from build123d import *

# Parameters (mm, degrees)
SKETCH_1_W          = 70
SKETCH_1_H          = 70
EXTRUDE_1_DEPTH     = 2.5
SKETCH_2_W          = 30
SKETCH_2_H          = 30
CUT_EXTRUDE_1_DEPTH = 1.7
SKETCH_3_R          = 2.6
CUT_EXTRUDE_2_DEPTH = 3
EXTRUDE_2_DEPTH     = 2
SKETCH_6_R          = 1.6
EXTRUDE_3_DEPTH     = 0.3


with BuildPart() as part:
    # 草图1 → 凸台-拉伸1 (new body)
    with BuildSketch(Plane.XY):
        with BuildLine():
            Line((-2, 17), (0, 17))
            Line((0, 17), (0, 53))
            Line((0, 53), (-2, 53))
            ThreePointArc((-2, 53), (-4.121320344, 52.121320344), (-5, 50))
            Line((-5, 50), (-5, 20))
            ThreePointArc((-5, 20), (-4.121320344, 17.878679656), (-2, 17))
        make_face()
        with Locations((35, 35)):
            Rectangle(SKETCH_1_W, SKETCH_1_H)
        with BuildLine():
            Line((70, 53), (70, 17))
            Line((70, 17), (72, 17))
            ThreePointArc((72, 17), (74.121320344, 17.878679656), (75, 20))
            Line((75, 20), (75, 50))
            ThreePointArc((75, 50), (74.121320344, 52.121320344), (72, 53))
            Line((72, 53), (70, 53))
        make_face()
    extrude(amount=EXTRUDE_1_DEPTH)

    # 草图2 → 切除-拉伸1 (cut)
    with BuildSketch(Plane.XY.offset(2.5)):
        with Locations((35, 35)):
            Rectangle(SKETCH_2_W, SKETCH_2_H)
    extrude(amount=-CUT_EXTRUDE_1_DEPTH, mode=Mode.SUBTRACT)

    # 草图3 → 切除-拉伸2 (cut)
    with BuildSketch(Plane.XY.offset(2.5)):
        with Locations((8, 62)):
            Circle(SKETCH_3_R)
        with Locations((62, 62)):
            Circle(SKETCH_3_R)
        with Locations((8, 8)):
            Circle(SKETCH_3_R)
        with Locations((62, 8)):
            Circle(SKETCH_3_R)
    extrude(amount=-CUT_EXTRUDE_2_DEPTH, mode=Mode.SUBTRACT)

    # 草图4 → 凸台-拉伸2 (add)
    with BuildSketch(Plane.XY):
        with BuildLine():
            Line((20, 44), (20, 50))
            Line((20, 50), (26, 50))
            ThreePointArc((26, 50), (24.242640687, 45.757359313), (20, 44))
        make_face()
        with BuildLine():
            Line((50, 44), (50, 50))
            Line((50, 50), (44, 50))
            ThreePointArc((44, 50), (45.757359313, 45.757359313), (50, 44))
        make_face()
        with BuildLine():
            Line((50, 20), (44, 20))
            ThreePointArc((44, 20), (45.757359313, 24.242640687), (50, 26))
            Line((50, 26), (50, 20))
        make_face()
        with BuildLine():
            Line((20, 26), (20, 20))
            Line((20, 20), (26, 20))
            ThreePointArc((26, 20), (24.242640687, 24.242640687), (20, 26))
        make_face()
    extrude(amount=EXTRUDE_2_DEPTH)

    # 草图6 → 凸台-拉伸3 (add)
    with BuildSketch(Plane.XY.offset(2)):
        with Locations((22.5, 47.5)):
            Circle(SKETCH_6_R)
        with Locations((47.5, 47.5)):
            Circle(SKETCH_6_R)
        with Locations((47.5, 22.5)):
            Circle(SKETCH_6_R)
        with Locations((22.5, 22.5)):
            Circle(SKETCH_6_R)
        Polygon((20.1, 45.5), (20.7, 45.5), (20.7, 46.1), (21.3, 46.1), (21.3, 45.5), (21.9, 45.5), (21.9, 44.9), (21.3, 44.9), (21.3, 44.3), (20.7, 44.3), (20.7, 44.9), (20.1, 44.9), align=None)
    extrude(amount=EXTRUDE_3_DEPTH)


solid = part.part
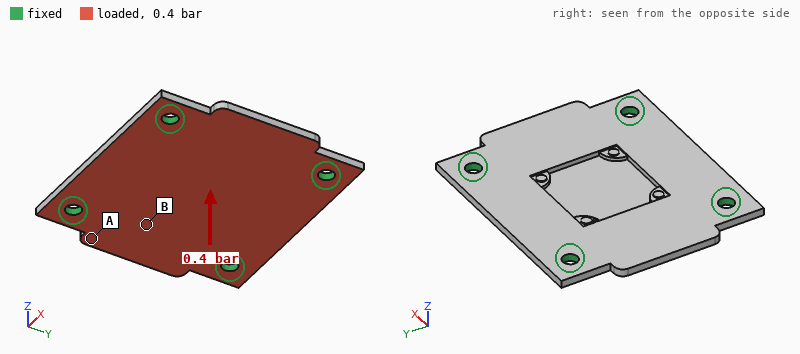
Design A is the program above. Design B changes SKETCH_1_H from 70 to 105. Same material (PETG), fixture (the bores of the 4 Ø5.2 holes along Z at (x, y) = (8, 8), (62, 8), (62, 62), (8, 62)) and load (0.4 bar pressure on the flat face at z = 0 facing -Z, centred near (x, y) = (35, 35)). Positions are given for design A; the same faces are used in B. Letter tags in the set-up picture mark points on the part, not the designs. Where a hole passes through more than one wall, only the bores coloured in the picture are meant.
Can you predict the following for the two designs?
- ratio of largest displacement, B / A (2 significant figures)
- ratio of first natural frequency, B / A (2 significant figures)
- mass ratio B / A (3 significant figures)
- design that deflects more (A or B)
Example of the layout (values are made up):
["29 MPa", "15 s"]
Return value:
["0.87", "0.69", "1.53", "A"]
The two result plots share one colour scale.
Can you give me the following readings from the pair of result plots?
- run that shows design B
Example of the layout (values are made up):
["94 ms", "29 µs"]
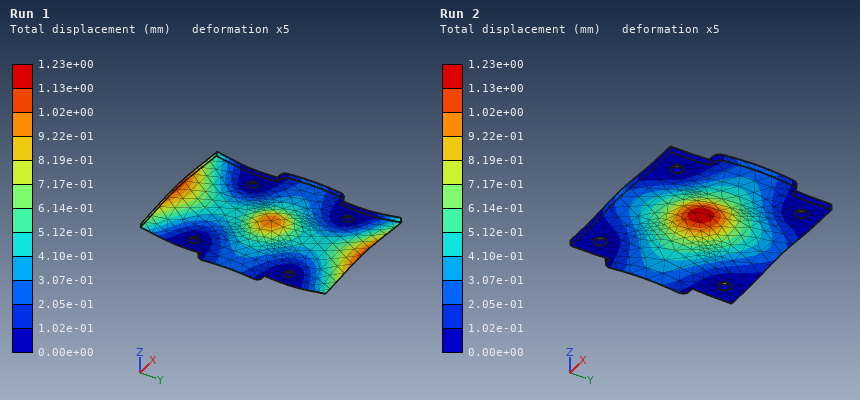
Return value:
["Run 1"]
